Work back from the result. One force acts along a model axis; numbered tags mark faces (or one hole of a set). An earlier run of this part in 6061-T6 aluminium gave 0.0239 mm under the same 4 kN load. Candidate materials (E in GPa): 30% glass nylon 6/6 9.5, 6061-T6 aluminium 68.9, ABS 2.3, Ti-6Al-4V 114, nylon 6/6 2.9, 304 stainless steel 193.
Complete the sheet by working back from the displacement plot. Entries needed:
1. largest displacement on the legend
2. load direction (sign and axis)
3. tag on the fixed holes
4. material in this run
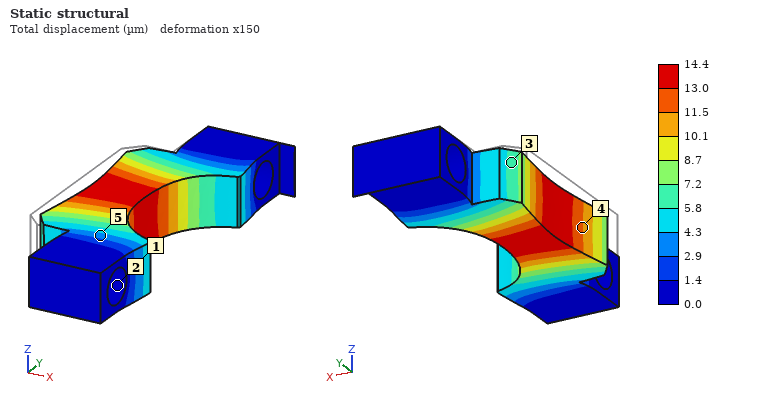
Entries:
14.4 µm
+X
2
Ti-6Al-4V
